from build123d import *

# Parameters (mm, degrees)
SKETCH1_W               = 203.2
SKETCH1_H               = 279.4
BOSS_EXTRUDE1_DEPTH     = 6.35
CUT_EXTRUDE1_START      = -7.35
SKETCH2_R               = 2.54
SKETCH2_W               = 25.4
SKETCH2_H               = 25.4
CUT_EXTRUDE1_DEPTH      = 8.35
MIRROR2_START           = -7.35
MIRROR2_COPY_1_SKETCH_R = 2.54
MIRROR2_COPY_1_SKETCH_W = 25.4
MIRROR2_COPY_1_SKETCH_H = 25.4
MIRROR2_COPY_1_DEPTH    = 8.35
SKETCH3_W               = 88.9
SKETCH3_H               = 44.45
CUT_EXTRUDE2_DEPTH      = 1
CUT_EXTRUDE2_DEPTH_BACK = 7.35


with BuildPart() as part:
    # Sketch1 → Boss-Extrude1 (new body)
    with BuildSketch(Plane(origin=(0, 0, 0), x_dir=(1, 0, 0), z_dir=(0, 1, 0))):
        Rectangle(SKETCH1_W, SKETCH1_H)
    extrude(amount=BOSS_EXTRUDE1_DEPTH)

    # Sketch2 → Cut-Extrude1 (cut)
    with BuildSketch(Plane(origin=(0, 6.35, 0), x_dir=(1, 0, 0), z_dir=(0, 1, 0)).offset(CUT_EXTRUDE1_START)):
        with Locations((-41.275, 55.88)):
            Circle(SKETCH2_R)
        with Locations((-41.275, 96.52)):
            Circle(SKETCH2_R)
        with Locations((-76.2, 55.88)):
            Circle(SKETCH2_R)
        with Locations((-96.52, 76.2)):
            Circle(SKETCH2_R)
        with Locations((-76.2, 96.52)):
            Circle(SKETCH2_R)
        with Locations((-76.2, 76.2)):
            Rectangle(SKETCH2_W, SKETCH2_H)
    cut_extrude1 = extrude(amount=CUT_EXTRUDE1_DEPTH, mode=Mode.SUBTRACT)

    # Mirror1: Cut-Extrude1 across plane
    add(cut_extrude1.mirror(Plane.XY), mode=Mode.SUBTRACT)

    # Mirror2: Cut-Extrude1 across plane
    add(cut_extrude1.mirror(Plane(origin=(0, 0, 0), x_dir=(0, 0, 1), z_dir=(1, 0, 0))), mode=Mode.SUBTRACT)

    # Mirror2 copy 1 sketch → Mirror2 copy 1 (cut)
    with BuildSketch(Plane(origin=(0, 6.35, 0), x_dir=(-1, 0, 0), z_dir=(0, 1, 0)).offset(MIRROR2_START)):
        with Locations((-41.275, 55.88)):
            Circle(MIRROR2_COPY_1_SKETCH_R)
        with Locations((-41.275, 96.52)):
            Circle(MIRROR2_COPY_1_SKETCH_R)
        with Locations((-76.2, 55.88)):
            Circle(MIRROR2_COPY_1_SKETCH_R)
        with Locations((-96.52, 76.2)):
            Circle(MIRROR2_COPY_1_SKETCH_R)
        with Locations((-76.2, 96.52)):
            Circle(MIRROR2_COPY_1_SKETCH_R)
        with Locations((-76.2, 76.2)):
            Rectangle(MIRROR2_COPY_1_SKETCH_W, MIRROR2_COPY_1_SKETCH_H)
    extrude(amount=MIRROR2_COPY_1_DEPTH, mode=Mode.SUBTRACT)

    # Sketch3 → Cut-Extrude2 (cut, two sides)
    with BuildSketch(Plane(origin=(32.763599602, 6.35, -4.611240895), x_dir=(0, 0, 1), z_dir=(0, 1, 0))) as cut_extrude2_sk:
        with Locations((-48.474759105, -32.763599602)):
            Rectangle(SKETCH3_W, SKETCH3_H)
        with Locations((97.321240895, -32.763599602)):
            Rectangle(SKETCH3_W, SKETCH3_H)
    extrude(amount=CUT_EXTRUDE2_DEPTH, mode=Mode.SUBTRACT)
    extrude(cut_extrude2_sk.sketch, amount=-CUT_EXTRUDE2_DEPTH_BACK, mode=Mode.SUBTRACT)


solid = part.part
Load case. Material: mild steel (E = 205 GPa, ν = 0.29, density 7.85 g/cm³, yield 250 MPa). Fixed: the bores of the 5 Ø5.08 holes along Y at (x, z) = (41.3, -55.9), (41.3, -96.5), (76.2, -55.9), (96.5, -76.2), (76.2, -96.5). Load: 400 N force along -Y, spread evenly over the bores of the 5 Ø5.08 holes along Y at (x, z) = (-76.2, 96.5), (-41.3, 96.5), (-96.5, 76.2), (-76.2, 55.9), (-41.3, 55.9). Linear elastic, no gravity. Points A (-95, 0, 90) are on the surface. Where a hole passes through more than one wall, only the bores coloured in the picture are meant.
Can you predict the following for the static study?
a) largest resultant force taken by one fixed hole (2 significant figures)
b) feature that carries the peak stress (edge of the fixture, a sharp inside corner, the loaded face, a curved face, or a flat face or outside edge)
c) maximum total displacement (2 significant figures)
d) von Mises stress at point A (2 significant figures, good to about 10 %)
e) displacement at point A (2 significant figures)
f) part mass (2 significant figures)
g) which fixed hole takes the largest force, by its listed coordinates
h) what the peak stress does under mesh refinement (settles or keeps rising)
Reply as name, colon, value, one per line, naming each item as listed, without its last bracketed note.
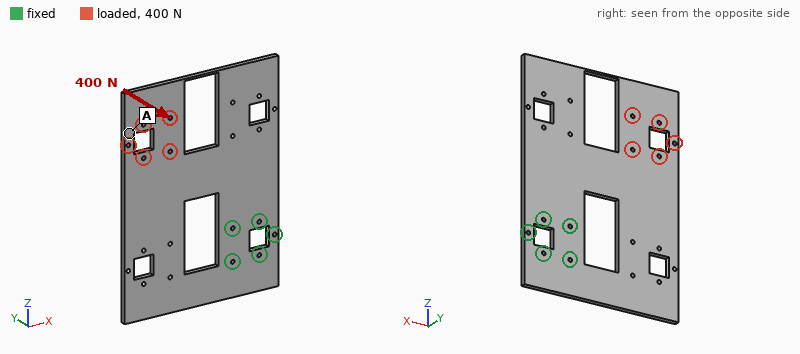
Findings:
largest resultant force taken by one fixed hole: 1.3 kN
feature that carries the peak stress: edge of the fixture
maximum total displacement: 2.5 mm
von Mises stress at point A: 16 MPa
displacement at point A: 2.0 mm
part mass: 2.3 kg
which fixed hole takes the largest force, by its listed coordinates: (41.3, -55.9)
what the peak stress does under mesh refinement: keeps rising
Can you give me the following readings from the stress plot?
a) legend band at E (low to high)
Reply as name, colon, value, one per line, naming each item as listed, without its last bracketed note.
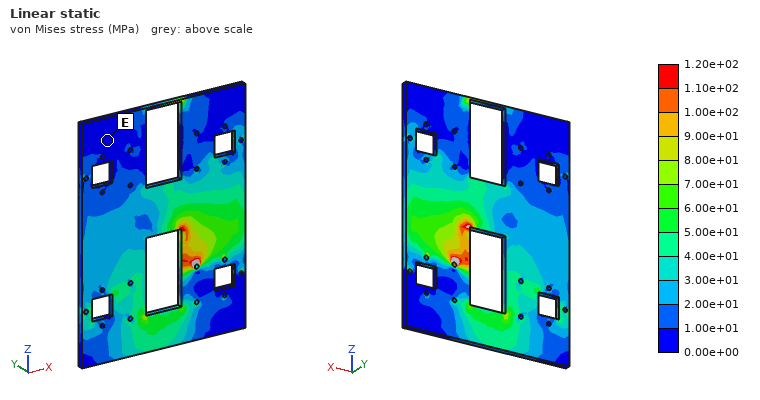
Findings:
legend band at E: 0.00e+00 to 1.00e+01 MPa
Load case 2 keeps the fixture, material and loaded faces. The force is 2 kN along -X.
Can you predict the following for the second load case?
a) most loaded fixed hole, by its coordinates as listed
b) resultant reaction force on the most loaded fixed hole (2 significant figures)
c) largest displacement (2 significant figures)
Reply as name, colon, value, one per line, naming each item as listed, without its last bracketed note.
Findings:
most loaded fixed hole, by its coordinates as listed: (41.3, -55.9)
resultant reaction force on the most loaded fixed hole: 3.3 kN
largest displacement: 53 µm
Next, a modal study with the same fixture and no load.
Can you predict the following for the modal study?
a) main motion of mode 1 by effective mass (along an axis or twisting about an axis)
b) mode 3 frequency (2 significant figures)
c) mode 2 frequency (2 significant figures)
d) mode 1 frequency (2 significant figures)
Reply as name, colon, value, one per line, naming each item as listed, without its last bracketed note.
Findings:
main motion of mode 1 by effective mass: along Y
mode 3 frequency: 320 Hz
mode 2 frequency: 170 Hz
mode 1 frequency: 98 Hz
